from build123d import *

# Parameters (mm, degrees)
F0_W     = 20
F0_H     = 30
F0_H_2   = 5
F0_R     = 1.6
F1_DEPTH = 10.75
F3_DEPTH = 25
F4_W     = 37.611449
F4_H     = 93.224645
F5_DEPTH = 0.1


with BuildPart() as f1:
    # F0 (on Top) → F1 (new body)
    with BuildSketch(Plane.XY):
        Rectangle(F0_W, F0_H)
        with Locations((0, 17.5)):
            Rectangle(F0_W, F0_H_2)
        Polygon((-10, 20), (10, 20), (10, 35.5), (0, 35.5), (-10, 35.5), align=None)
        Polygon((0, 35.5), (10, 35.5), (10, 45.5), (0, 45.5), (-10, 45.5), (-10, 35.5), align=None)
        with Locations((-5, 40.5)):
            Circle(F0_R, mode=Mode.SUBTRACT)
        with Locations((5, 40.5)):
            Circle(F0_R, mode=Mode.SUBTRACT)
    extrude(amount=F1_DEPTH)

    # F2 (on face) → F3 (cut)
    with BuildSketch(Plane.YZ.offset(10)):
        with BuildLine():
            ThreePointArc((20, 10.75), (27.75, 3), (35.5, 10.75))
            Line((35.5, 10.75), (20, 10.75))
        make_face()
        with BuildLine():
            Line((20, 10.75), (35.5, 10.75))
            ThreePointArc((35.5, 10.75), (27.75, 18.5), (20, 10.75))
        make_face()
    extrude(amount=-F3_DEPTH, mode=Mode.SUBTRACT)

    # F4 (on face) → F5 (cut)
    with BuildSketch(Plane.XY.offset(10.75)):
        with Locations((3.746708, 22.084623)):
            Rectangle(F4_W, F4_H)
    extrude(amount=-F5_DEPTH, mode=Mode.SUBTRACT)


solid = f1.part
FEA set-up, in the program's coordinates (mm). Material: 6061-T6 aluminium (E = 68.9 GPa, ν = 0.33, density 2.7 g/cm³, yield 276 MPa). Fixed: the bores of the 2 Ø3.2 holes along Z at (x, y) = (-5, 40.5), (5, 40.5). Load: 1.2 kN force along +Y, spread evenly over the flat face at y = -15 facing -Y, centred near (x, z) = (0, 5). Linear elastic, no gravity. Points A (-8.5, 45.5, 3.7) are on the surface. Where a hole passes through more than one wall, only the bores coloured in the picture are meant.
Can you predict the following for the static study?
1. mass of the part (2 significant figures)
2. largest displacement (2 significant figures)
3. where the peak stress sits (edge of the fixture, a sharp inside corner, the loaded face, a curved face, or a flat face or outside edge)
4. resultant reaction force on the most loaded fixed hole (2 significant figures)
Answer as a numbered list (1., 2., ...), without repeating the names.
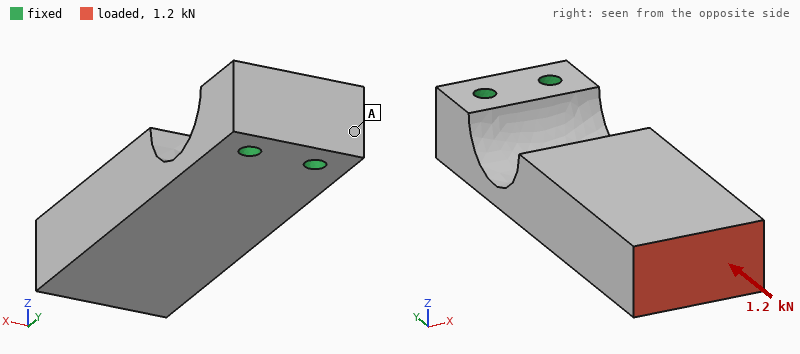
1. 29 g
2. 0.47 mm
3. a curved face
4. 610 N
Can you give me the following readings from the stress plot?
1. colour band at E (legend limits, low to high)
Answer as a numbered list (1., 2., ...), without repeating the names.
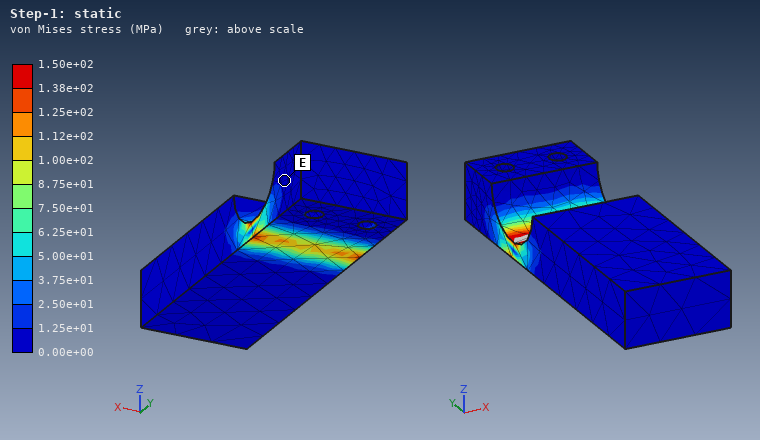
1. 0.00e+00 to 1.25e+01 MPa
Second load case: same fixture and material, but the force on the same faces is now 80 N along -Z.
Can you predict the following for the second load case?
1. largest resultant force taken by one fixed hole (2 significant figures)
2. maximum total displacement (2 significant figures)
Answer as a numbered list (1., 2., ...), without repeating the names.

1. 41 N
2. 0.40 mm
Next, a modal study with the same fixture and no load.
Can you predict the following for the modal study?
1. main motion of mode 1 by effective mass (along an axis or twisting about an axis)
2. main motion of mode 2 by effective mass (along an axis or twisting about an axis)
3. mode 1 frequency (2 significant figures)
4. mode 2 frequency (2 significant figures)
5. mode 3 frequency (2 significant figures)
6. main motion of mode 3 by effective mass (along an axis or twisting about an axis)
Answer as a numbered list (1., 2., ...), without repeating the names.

1. along Z
2. along X
3. 780 Hz
4. 2900 Hz
5. 5500 Hz
6. twisting about Y
